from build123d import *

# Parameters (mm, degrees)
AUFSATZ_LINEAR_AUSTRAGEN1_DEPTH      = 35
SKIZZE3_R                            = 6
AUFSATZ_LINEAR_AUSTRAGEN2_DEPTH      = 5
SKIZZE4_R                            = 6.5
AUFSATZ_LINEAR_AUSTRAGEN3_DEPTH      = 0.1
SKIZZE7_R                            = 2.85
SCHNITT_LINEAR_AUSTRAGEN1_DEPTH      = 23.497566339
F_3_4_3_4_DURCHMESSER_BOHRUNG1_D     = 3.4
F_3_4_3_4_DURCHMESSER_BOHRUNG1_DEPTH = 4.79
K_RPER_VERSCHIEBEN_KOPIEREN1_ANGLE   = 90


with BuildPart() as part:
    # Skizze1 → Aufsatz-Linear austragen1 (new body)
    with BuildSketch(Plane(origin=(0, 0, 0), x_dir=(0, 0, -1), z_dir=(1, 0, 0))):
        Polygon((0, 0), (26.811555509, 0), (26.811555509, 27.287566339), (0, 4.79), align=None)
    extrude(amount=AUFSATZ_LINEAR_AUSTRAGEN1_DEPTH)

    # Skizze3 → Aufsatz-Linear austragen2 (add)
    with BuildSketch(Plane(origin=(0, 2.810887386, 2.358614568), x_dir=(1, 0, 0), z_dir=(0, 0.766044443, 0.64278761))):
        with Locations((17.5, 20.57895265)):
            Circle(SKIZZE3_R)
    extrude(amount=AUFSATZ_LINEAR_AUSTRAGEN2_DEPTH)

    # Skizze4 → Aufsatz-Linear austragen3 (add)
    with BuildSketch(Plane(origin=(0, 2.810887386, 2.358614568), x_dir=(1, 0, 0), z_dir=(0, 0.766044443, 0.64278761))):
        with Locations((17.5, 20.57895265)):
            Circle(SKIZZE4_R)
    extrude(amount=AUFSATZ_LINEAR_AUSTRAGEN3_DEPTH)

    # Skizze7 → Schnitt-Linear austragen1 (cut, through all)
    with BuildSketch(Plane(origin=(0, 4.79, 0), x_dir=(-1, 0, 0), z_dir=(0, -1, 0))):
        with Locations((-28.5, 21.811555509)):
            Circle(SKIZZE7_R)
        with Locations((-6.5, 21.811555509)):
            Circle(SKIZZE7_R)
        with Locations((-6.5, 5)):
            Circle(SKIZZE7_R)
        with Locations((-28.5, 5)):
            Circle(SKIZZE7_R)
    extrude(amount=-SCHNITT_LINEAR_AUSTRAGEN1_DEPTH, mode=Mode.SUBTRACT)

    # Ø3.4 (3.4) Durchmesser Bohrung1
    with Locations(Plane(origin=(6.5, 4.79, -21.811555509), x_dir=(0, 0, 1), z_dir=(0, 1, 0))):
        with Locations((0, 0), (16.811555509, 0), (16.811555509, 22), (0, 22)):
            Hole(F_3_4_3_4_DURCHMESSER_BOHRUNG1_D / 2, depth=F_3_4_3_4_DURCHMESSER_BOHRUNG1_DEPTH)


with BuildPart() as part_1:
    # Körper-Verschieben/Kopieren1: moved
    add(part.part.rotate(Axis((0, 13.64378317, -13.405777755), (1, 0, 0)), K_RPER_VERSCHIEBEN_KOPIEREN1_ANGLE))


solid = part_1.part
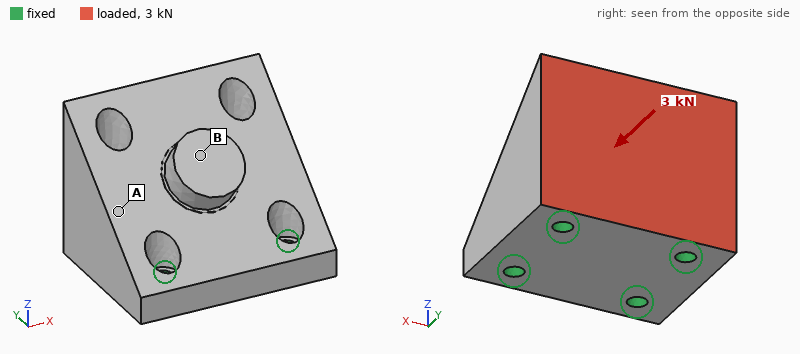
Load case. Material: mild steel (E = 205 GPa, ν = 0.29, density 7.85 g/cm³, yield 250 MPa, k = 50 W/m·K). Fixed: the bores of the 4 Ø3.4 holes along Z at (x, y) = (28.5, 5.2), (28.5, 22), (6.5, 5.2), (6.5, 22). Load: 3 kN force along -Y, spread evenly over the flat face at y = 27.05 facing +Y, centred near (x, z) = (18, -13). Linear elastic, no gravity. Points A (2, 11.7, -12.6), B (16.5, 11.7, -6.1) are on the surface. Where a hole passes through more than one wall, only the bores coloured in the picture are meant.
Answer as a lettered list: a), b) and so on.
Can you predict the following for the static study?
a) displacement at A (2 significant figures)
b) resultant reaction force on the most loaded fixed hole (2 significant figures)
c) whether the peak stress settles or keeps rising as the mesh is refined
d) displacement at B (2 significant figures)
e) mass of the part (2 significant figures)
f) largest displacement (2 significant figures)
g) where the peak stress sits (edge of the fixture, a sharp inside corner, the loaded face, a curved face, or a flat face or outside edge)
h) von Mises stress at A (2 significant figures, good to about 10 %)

a) 1.6 µm
b) 1.2 kN
c) keeps rising
d) 2.9 µm
e) 110 g
f) 6.4 µm
g) edge of the fixture
h) 14 MPa
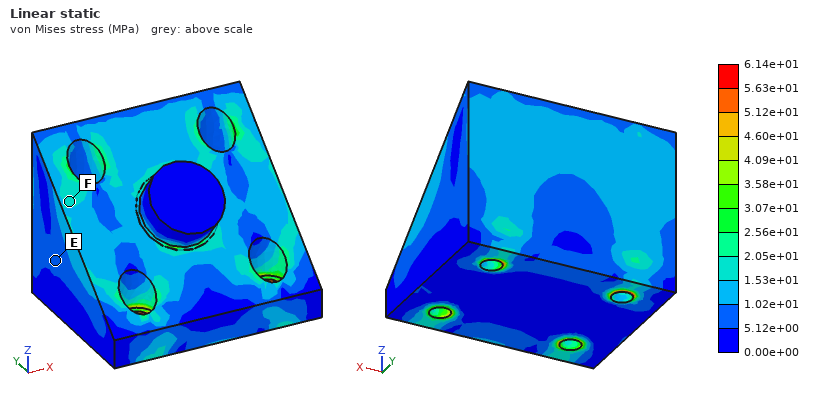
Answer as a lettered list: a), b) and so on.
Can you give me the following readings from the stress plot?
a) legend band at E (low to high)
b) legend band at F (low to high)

a) 5.12e+00 to 1.02e+01 MPa
b) 1.53e+01 to 2.05e+01 MPa
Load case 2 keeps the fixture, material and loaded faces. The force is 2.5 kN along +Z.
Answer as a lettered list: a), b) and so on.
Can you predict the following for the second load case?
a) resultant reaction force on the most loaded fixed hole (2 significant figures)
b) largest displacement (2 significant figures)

a) 1.5 kN
b) 4.9 µm
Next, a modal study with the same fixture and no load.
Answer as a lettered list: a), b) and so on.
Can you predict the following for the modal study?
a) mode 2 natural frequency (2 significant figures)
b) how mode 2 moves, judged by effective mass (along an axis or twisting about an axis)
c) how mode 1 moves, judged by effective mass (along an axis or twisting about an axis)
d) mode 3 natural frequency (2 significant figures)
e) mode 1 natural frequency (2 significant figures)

a) 23 kHz
b) along X
c) along Y
d) 34 kHz
e) 21 kHz
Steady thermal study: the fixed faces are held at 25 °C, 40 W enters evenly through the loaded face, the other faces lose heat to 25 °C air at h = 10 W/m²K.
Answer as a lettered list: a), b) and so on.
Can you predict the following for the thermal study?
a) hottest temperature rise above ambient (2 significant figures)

a) 38 K
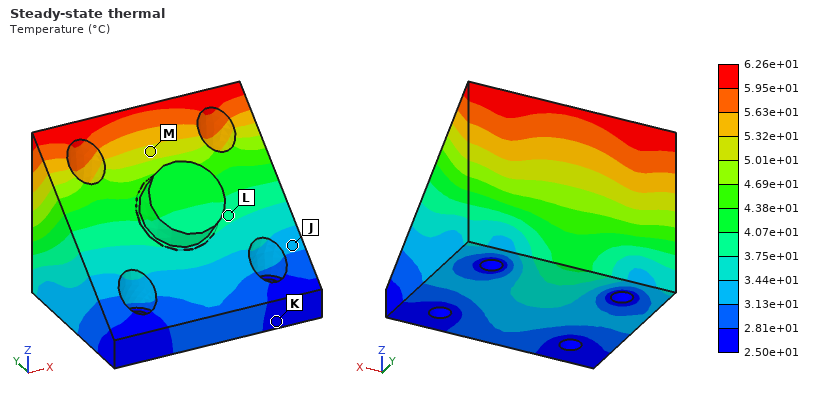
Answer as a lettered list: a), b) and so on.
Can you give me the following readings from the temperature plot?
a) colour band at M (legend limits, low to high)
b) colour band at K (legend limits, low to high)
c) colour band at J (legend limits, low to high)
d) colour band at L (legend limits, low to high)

a) 5.01e+01 to 5.32e+01 °C
b) 2.50e+01 to 2.81e+01 °C
c) 3.13e+01 to 3.44e+01 °C
d) 3.75e+01 to 4.07e+01 °C
